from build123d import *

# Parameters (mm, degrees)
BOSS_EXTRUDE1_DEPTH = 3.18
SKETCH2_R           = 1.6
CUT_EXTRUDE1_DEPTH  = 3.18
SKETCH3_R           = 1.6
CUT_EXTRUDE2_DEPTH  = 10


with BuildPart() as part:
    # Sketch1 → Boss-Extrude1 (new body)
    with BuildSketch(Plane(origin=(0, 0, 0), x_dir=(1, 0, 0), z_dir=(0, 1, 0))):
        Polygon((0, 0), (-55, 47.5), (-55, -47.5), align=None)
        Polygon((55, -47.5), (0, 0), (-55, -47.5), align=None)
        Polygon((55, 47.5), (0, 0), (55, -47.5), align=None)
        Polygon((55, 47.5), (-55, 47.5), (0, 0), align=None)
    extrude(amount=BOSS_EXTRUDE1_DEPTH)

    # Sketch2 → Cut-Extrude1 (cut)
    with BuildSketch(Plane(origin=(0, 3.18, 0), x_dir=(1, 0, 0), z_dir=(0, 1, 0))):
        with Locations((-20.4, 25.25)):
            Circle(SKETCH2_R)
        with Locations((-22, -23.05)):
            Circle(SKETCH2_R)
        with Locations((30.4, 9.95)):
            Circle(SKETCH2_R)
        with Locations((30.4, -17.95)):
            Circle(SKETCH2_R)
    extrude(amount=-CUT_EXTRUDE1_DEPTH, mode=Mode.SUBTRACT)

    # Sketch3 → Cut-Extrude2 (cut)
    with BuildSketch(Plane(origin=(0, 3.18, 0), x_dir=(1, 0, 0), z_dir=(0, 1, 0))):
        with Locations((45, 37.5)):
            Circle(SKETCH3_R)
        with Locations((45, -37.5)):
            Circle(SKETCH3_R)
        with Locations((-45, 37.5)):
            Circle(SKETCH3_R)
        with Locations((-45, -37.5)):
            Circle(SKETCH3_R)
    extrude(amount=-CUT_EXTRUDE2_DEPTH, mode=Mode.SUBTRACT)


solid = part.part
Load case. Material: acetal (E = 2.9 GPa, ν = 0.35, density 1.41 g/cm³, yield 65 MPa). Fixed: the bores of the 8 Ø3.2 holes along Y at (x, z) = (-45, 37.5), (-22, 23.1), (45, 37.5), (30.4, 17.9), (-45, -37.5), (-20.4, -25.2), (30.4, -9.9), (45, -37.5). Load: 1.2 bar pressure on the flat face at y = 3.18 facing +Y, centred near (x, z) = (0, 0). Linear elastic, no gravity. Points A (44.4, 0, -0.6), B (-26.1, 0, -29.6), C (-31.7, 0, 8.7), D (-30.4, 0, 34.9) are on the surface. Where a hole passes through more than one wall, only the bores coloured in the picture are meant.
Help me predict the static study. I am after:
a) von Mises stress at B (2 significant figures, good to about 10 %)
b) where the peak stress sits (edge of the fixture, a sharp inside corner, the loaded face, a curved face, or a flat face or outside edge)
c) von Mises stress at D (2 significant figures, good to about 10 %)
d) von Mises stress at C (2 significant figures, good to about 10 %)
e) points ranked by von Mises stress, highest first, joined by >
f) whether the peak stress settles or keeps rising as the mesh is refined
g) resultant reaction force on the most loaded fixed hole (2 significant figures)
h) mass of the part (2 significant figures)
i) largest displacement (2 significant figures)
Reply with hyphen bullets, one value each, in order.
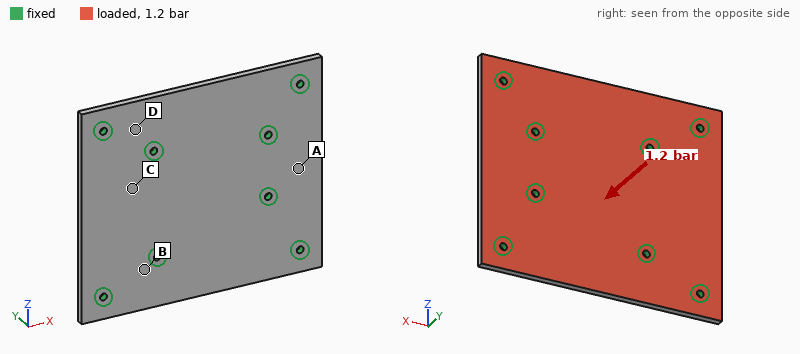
- 14 MPa
- edge of the fixture
- 11 MPa
- 6.3 MPa
- B > D > C > A
- keeps rising
- 250 N
- 47 g
- 1.0 mm
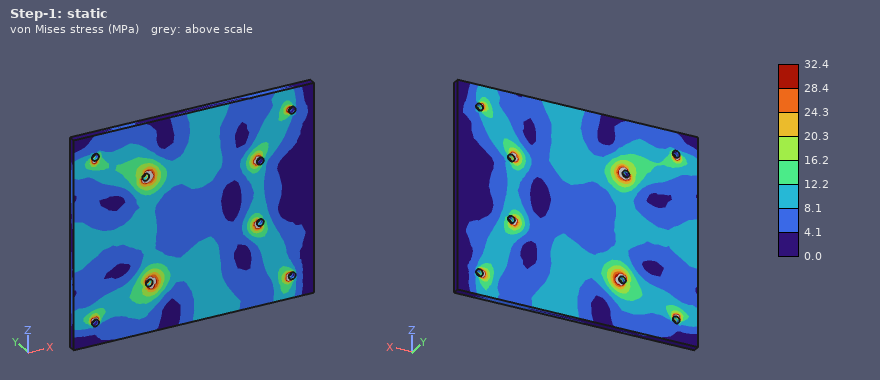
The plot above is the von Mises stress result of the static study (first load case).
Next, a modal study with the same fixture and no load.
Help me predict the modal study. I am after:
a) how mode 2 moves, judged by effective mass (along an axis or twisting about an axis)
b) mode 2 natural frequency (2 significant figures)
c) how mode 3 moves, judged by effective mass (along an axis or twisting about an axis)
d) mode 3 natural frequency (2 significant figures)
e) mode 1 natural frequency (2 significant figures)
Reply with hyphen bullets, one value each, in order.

- twisting about X
- 1000 Hz
- along Y
- 1100 Hz
- 990 Hz
